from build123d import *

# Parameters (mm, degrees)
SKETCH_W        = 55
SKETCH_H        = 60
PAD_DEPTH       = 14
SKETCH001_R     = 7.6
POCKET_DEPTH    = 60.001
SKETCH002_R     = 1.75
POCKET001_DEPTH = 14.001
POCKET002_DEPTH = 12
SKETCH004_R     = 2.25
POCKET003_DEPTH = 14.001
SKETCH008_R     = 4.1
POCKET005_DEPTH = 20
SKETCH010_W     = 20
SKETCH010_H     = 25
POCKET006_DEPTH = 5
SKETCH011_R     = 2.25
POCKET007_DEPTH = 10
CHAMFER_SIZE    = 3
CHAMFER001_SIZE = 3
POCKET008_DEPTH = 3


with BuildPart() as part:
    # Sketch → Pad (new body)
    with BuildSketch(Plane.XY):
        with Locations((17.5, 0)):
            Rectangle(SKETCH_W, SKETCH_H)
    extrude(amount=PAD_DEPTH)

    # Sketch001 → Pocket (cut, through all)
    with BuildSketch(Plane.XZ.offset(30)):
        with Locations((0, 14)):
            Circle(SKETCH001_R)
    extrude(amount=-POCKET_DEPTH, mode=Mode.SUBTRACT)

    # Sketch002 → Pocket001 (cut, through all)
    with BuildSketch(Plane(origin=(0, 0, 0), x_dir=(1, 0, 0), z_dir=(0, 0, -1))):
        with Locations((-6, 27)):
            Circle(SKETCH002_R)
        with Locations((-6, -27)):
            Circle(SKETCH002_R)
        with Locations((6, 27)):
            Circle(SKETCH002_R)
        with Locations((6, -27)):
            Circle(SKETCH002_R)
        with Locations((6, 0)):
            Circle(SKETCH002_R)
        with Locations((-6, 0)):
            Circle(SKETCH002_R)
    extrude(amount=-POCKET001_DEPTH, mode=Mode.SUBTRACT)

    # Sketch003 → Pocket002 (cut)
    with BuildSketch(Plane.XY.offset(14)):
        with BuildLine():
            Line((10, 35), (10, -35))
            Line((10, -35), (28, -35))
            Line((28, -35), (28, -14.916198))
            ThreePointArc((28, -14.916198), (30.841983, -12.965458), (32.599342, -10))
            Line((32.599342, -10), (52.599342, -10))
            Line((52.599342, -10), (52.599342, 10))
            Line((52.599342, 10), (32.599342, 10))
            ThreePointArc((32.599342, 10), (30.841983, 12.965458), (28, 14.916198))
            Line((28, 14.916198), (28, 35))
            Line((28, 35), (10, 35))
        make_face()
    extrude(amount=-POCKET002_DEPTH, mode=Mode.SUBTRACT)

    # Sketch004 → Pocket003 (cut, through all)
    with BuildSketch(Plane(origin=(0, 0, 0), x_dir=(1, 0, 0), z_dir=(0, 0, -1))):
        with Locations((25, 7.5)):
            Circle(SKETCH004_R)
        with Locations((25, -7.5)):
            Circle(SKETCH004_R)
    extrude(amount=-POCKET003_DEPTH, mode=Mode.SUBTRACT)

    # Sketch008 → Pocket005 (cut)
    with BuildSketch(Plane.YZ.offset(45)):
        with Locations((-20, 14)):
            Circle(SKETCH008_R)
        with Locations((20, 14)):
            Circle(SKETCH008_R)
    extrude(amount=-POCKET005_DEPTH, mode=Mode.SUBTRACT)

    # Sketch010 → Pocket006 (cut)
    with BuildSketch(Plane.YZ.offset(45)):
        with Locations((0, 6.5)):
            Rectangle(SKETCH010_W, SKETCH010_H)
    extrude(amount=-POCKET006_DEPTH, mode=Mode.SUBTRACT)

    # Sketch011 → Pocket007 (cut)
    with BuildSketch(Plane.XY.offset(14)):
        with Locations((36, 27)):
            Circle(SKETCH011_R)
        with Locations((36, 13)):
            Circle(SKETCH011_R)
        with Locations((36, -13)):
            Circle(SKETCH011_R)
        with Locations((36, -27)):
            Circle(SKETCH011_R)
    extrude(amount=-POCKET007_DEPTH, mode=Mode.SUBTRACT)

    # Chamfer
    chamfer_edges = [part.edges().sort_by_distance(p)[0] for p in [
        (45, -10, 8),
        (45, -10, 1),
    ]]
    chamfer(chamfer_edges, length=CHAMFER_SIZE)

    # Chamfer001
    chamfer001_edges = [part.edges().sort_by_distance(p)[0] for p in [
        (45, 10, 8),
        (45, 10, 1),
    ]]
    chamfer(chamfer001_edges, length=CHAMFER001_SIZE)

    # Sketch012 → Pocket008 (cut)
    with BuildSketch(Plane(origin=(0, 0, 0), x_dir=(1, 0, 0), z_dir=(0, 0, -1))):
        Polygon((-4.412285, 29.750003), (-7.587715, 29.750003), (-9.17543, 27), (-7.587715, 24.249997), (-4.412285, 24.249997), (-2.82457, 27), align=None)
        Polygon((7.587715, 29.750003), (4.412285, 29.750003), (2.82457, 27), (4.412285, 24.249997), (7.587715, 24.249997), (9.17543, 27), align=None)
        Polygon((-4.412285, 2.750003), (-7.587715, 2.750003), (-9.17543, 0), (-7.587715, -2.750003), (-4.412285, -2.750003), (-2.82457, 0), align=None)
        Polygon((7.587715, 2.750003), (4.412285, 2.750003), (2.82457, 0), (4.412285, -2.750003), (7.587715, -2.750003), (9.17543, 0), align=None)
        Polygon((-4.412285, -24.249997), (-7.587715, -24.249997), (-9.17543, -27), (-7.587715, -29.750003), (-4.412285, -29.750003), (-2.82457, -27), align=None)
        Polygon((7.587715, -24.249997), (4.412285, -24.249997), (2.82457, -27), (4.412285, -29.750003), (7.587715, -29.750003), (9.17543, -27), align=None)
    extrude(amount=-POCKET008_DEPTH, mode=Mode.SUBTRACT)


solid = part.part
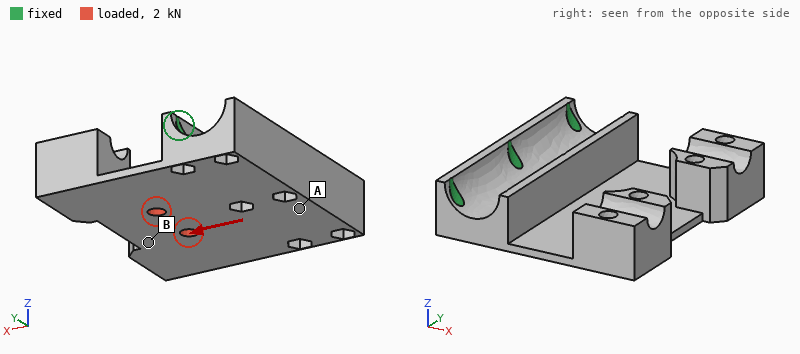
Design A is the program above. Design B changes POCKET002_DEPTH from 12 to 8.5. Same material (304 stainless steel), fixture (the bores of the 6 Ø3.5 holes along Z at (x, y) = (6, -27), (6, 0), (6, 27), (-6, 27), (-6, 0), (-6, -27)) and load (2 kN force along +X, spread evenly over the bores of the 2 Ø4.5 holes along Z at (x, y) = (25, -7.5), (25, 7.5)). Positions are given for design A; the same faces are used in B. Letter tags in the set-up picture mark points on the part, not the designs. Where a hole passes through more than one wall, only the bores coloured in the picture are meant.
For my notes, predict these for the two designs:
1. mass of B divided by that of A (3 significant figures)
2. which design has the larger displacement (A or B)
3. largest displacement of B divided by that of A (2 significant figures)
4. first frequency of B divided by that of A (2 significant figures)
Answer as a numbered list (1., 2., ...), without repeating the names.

1. 1.22
2. A
3. 0.33
4. 3.7
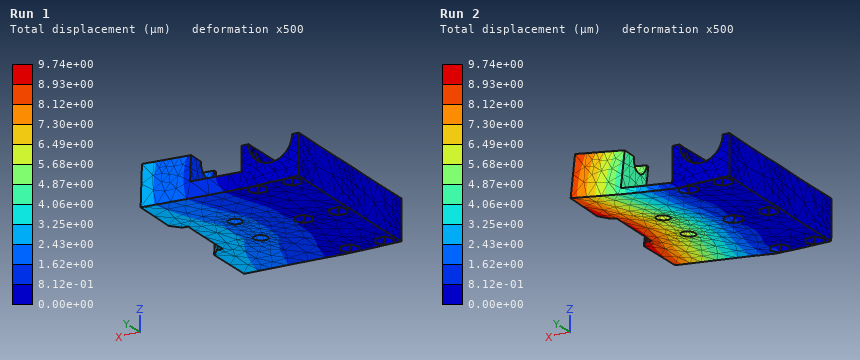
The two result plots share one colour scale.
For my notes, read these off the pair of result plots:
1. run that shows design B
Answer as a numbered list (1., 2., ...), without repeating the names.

1. Run 1
